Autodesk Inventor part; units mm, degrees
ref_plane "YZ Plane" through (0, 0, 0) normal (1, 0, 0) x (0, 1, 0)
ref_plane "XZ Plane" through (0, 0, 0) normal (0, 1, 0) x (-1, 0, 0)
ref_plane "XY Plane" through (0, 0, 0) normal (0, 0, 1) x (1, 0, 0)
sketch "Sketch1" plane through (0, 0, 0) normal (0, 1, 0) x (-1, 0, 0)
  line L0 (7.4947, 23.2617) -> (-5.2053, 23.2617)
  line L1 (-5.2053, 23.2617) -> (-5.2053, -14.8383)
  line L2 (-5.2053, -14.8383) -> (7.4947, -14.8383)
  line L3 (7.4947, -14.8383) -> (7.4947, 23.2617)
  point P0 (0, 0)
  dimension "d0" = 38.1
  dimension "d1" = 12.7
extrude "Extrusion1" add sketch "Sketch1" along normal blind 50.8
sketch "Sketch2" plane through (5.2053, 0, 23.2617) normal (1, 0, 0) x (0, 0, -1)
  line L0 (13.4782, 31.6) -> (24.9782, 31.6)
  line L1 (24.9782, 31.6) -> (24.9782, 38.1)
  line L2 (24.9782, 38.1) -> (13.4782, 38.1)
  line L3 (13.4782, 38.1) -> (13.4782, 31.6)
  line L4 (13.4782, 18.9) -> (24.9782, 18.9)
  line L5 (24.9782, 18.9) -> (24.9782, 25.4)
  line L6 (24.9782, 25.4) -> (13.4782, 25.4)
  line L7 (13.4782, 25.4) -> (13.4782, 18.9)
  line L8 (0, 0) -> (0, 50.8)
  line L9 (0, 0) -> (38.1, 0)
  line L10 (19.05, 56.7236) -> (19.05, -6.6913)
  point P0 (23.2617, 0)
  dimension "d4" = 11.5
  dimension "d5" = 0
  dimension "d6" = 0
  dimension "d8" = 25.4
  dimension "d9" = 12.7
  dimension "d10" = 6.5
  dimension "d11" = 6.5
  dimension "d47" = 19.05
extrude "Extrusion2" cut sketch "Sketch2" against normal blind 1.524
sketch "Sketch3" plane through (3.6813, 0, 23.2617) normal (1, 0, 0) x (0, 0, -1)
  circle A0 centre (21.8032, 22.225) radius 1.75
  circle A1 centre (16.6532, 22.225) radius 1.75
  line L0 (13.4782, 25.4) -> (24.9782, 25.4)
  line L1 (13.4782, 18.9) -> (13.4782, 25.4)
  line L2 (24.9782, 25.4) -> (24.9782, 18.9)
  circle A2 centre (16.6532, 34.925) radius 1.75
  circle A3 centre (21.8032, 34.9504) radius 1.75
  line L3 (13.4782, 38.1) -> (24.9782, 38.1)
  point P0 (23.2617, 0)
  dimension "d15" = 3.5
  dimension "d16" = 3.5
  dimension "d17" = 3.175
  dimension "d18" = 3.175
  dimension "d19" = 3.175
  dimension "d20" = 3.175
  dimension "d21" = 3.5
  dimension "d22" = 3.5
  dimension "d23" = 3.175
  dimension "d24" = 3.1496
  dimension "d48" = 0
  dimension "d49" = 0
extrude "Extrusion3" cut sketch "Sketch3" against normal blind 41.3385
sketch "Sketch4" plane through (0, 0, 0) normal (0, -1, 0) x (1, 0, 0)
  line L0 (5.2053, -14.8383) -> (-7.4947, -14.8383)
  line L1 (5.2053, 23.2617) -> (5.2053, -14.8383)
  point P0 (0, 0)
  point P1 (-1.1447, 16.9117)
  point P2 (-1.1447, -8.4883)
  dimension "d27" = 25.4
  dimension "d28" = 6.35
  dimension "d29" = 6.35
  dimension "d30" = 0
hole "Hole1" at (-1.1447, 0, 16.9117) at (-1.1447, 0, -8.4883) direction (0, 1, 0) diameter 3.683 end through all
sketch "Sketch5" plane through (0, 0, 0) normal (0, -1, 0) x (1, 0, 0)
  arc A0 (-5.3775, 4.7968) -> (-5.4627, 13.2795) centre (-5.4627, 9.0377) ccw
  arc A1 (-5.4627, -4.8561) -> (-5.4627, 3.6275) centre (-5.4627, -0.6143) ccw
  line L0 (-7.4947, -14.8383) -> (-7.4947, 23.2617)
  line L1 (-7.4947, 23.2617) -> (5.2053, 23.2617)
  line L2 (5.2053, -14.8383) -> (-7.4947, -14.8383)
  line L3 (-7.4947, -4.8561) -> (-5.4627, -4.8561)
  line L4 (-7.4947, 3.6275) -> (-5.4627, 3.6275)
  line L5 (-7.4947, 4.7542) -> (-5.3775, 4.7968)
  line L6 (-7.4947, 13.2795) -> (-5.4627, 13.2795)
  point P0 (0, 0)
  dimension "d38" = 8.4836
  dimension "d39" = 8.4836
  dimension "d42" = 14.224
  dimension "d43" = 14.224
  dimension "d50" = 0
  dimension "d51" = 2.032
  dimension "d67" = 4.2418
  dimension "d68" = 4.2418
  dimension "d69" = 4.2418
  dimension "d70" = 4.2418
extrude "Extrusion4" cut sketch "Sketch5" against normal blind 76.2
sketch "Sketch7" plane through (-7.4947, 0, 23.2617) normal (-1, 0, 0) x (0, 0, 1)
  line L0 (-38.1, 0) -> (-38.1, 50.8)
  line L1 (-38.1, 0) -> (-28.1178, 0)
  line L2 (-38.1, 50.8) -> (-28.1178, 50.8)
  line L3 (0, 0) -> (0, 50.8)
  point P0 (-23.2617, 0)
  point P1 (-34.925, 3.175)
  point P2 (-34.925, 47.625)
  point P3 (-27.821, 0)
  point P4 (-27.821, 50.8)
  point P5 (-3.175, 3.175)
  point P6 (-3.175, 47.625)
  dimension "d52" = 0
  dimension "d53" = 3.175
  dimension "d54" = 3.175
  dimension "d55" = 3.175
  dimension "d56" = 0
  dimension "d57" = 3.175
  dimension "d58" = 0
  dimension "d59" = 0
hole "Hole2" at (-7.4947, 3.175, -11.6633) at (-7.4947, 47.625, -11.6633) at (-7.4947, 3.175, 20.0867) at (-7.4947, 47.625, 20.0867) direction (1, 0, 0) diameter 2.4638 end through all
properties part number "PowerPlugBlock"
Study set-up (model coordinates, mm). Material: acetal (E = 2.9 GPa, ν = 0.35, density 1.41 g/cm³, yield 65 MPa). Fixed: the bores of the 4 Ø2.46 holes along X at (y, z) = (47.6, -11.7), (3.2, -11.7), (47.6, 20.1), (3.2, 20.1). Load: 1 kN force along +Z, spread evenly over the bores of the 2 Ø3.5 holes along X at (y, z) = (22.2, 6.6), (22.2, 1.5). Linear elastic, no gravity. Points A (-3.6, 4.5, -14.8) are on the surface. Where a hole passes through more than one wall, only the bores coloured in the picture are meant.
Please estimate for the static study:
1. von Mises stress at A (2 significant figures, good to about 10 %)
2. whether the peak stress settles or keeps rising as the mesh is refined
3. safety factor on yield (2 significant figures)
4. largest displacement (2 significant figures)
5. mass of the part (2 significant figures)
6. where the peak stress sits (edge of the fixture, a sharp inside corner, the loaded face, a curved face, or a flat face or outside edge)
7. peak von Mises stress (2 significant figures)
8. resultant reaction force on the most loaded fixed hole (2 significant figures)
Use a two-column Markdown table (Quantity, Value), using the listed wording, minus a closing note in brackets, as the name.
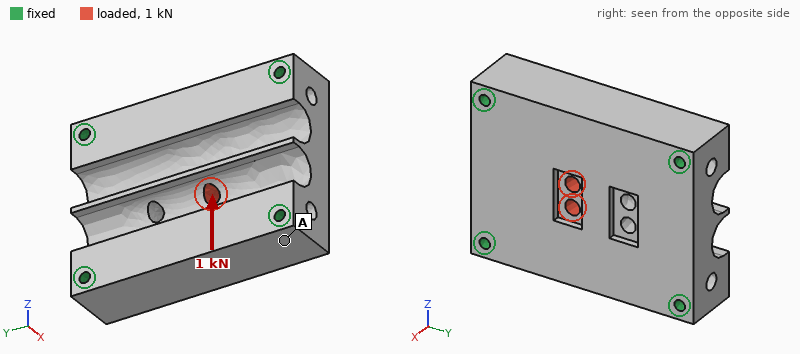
| Quantity | Value |
|---|---|
| von Mises stress at A | 3.2 MPa |
| whether the peak stress settles or keeps rising as the mesh is refined | settles |
| safety factor on yield | 2.5 |
| largest displacement | 95 µm |
| mass of the part | 26 g |
| where the peak stress sits | the loaded face |
| peak von Mises stress | 26 MPa |
| resultant reaction force on the most loaded fixed hole | 350 N |
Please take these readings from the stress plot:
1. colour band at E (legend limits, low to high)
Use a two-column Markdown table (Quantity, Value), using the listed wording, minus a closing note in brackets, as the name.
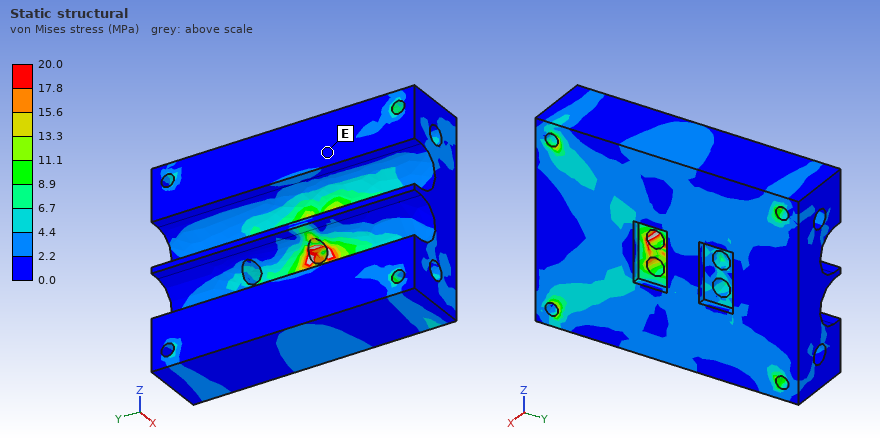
| Quantity | Value |
|---|---|
| colour band at E | 0.0 to 2.2 MPa |
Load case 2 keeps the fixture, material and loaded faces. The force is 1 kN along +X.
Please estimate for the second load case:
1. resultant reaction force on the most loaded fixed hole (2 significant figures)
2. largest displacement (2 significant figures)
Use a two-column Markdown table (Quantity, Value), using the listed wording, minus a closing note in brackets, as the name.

| Quantity | Value |
|---|---|
| resultant reaction force on the most loaded fixed hole | 320 N |
| largest displacement | 0.23 mm |
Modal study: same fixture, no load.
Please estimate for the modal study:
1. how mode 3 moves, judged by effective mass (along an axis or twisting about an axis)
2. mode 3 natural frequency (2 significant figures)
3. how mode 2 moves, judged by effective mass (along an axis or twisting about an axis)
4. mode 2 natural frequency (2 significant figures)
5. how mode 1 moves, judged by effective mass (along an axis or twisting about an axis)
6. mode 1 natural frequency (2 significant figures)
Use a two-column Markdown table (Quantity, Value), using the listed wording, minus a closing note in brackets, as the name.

| Quantity | Value |
|---|---|
| how mode 3 moves, judged by effective mass | along Z |
| mode 3 natural frequency | 7300 Hz |
| how mode 2 moves, judged by effective mass | along Z |
| mode 2 natural frequency | 6200 Hz |
| how mode 1 moves, judged by effective mass | along X |
| mode 1 natural frequency | 4900 Hz |
